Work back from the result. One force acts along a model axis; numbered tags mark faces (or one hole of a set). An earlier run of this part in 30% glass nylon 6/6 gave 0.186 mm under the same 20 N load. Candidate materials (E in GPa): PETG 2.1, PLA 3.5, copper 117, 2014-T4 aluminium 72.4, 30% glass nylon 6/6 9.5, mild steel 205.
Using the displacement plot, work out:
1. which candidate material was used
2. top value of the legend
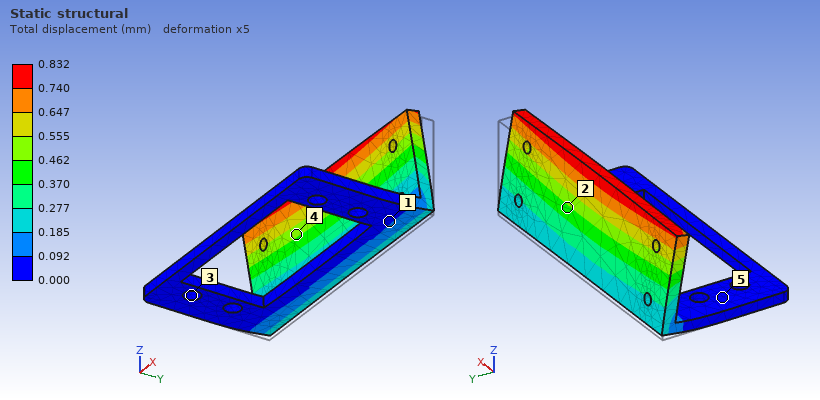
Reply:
PETG
0.832 mm
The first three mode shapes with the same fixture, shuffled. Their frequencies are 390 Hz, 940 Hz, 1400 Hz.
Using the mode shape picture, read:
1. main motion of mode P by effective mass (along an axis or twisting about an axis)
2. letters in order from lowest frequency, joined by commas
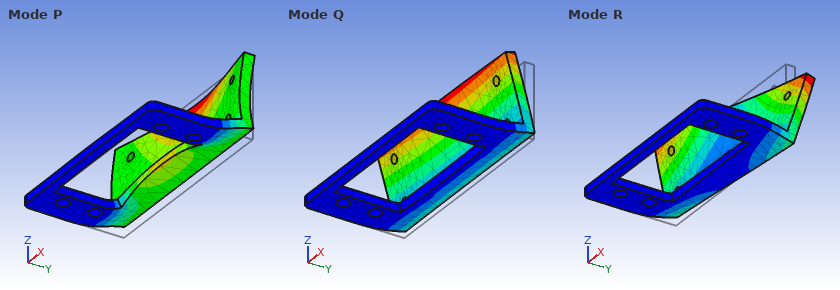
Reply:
along Z
Q, R, P
